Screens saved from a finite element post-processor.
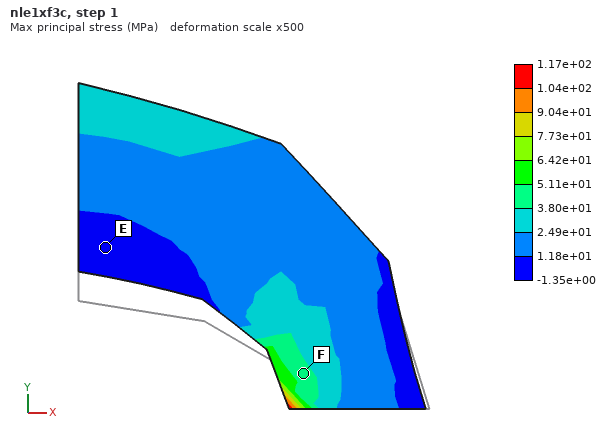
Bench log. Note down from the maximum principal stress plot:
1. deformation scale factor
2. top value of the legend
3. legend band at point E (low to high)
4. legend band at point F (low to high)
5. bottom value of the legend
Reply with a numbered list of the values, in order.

1. 500
2. 1.17e+02 MPa
3. -1.35e+00 to 1.18e+01 MPa
4. 3.80e+01 to 5.11e+01 MPa
5. -1.35e+00 MPa
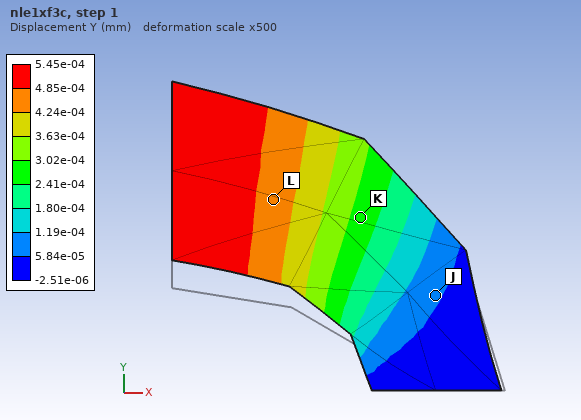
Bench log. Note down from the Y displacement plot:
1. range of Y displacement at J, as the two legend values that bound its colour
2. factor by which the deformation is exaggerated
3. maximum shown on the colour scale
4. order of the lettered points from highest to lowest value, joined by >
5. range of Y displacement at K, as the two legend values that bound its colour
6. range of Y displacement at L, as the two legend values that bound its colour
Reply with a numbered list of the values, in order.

1. 5.84e-05 to 1.19e-04 mm
2. 500
3. 5.45e-04 mm
4. L > K > J
5. 2.41e-04 to 3.02e-04 mm
6. 4.24e-04 to 4.85e-04 mm
